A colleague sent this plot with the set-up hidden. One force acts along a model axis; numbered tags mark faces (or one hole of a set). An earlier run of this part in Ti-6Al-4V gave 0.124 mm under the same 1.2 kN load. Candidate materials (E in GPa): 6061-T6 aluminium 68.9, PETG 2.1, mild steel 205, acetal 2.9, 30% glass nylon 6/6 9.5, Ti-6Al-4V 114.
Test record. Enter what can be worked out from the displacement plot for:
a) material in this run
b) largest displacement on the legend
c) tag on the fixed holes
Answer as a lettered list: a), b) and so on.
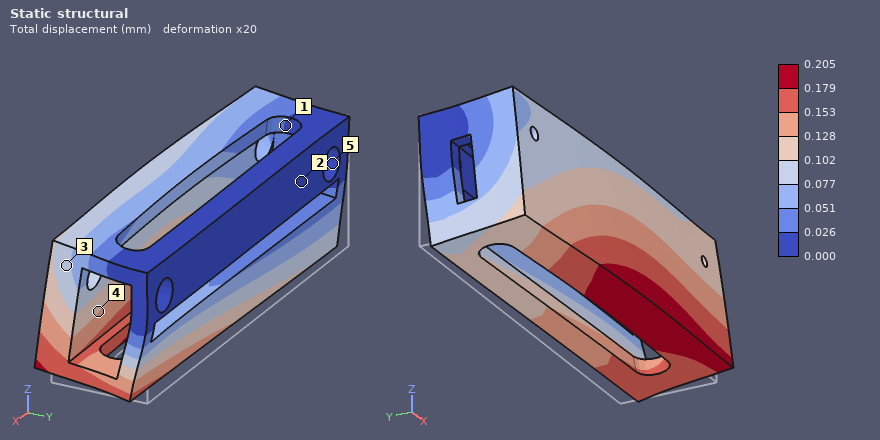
a) 6061-T6 aluminium
b) 0.205 mm
c) 5
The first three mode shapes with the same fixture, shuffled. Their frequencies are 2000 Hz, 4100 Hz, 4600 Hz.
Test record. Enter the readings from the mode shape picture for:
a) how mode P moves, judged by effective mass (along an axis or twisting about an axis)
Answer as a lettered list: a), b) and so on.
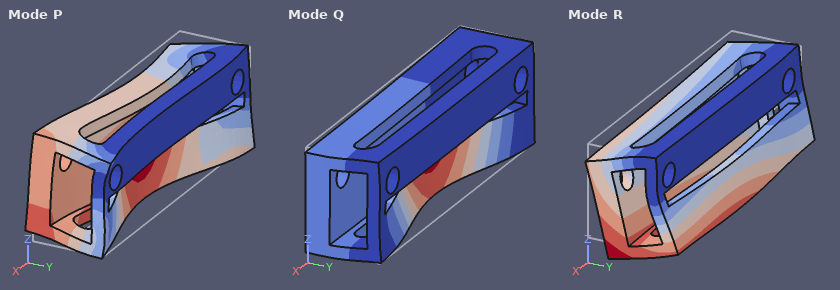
a) along X
